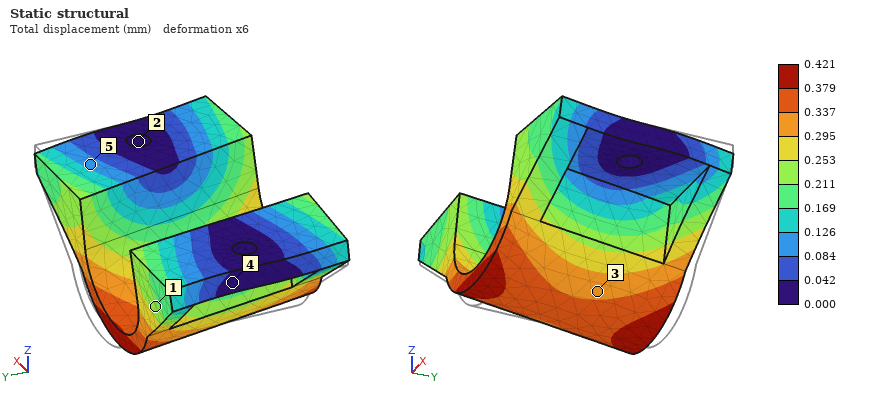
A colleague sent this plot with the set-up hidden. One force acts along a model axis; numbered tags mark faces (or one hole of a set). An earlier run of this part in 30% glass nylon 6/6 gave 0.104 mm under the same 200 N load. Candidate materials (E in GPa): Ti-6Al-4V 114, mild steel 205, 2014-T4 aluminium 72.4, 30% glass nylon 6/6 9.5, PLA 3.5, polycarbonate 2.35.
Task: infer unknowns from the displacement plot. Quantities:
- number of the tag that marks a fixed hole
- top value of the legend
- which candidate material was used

2
0.421 mm
polycarbonate
